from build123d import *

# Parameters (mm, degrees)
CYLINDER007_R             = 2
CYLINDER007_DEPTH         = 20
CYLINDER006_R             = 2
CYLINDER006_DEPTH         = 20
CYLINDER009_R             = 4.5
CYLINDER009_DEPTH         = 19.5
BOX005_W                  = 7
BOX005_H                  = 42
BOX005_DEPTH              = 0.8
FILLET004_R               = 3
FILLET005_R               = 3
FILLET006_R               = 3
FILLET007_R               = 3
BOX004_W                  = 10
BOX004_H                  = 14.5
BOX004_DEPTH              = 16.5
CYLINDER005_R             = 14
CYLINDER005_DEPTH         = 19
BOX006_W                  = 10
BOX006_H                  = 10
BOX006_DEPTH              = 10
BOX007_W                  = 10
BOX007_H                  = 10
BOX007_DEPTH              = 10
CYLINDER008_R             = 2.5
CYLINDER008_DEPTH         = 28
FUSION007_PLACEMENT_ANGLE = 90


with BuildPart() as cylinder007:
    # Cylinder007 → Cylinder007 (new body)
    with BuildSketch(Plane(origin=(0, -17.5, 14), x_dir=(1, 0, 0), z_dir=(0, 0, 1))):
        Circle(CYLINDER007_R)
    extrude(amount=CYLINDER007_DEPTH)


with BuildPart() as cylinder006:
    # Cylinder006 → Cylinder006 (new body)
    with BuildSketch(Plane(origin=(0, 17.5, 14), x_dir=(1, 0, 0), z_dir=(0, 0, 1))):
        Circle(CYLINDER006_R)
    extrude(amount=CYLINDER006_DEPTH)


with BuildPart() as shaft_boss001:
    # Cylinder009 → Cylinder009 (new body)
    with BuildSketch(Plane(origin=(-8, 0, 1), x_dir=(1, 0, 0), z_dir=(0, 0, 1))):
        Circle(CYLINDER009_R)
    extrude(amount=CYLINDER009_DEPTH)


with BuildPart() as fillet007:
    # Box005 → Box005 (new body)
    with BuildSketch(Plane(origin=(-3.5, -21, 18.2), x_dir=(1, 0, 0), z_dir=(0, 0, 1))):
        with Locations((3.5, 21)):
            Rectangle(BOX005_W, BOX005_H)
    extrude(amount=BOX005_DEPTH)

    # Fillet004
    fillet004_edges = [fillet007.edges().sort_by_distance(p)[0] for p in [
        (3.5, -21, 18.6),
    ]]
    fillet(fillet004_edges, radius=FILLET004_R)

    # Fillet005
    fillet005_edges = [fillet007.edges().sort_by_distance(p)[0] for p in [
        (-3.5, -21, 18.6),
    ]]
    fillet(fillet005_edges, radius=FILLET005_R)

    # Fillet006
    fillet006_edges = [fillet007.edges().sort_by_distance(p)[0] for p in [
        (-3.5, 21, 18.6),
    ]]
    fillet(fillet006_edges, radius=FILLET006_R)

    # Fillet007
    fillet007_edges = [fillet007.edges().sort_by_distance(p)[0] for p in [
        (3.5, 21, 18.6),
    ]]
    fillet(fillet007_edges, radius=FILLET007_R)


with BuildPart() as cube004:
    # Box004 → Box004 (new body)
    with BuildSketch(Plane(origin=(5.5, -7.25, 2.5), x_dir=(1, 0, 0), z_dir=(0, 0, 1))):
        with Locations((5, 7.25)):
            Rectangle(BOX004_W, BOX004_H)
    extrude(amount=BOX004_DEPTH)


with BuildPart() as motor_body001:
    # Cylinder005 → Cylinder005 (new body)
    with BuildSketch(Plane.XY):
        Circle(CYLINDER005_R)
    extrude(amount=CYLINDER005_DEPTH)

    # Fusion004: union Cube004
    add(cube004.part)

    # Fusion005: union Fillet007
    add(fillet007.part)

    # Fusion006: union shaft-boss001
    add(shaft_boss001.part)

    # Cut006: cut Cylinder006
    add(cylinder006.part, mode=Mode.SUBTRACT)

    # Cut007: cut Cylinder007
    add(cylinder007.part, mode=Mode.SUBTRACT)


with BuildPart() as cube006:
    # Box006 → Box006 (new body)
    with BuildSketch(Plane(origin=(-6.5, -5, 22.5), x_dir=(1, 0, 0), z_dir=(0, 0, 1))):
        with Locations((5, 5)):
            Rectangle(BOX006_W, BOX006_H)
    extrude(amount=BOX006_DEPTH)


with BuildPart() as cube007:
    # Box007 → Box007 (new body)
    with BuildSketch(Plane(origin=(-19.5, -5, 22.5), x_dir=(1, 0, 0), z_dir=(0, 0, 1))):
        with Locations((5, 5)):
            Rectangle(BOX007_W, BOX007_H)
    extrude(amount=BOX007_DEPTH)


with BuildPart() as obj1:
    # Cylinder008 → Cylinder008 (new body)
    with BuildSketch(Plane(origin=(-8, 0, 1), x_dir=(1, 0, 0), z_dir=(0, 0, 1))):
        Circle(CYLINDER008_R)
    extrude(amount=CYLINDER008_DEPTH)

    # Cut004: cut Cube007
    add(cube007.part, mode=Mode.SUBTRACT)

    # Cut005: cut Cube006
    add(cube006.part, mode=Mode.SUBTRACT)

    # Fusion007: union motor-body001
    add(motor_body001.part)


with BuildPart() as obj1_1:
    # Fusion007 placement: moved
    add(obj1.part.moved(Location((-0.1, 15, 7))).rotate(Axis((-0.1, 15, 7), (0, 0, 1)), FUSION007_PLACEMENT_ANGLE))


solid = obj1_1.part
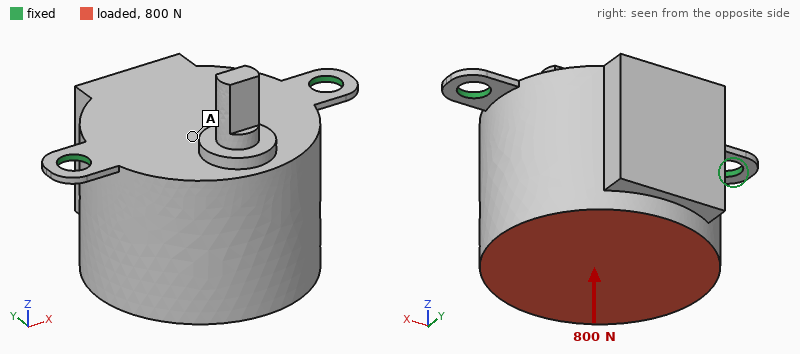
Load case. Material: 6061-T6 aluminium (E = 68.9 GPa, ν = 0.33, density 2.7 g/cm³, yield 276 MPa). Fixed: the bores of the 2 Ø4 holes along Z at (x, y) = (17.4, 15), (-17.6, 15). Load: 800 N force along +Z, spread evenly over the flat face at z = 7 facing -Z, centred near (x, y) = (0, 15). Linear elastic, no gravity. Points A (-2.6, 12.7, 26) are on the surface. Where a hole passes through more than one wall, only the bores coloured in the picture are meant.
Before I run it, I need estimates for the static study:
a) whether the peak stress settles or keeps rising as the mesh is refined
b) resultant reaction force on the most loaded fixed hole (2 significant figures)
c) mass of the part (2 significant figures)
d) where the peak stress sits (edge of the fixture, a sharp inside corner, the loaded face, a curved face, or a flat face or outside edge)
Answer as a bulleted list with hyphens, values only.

- keeps rising
- 470 N
- 34 g
- edge of the fixture
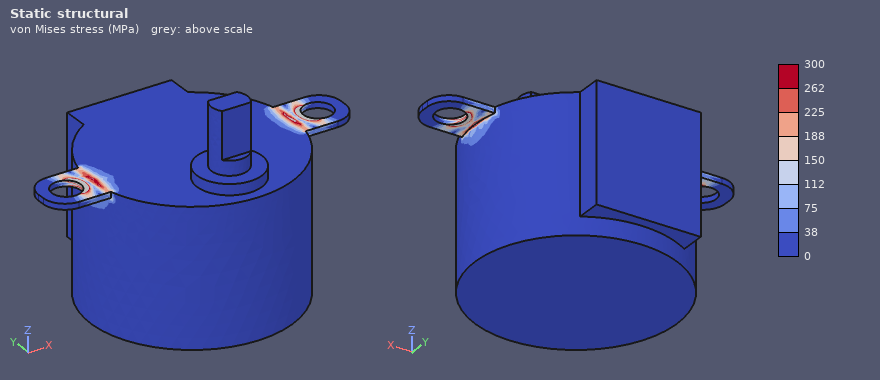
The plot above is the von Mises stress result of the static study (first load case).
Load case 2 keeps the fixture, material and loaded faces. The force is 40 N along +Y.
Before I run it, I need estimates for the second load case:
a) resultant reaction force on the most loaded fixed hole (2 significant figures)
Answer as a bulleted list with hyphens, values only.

- 20 N
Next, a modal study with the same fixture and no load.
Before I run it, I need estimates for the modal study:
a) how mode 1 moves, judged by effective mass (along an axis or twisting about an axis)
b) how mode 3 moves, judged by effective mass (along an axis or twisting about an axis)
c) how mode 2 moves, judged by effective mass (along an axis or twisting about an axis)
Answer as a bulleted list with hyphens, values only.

- along Y
- along X
- along Z
